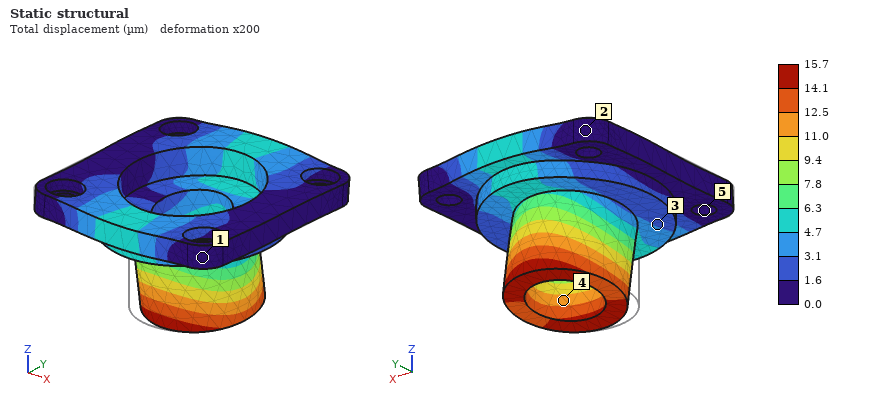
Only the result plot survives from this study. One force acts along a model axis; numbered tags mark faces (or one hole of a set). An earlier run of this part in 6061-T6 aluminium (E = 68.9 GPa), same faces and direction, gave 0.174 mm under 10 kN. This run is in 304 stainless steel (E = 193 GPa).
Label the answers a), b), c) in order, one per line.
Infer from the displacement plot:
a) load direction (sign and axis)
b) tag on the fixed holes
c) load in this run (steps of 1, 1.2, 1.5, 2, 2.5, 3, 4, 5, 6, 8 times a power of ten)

a) +Y
b) 5
c) 2.5 kN
